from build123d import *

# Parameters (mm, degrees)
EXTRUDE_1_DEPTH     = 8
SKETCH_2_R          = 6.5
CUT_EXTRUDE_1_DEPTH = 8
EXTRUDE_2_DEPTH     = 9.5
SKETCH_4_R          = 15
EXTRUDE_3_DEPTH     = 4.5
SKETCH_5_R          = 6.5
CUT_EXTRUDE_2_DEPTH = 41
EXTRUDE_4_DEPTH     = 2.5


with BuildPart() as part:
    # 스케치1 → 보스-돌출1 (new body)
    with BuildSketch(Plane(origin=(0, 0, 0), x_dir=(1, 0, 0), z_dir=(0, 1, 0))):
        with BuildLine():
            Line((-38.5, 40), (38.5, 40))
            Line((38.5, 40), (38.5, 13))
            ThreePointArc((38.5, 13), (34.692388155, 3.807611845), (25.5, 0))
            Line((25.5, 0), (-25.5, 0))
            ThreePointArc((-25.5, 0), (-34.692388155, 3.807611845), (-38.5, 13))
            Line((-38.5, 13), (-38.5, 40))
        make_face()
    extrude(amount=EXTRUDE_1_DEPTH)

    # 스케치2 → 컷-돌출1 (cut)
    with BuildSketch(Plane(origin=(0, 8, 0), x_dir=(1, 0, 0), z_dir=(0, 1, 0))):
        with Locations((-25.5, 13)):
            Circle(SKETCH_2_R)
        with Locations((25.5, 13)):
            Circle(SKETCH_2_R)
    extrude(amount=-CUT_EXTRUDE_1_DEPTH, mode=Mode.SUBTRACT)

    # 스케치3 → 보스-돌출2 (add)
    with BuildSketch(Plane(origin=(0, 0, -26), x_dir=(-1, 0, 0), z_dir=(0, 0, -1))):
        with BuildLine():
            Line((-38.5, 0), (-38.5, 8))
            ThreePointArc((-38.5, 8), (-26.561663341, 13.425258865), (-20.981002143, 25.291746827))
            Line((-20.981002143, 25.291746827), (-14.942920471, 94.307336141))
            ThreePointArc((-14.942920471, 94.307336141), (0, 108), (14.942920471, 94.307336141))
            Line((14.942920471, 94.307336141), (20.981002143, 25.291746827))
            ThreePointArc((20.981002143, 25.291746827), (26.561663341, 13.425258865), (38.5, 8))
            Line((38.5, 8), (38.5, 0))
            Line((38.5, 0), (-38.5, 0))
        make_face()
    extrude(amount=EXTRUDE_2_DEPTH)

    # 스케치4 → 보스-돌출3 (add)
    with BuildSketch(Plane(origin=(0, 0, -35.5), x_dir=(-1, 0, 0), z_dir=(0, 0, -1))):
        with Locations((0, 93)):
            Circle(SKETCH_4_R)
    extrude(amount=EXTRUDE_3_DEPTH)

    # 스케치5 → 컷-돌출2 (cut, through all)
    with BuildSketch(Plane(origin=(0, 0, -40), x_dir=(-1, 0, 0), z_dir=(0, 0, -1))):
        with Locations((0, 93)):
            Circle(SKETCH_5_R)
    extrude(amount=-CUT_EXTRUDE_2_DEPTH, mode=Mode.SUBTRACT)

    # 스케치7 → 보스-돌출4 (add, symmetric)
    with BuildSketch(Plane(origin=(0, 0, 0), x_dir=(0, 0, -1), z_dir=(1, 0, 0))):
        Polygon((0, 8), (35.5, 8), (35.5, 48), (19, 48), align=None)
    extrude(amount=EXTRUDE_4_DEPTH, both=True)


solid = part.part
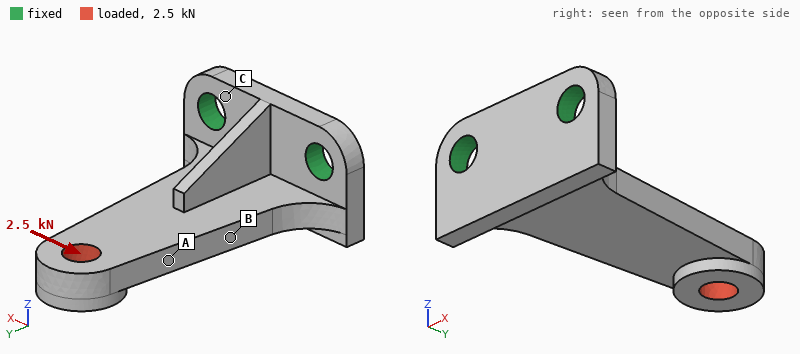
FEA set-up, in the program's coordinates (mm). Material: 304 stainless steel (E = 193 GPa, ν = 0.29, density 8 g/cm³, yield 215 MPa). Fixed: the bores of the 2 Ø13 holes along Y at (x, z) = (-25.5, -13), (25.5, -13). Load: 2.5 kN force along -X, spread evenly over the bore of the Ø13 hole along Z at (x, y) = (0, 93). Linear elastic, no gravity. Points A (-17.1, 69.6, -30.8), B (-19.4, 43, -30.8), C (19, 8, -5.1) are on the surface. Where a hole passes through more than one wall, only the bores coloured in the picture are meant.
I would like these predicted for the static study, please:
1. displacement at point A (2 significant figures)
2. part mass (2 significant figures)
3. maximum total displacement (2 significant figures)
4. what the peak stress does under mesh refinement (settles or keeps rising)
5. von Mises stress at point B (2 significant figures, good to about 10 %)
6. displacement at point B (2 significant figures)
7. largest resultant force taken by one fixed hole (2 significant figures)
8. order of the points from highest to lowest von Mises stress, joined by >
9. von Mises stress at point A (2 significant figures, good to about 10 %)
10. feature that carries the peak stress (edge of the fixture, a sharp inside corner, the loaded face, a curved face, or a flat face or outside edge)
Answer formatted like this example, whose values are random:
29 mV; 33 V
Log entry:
0.064 mm; 490 g; 0.12 mm; keeps rising; 54 MPa; 0.034 mm; 4.7 kN; B > A > C; 33 MPa; edge of the fixture
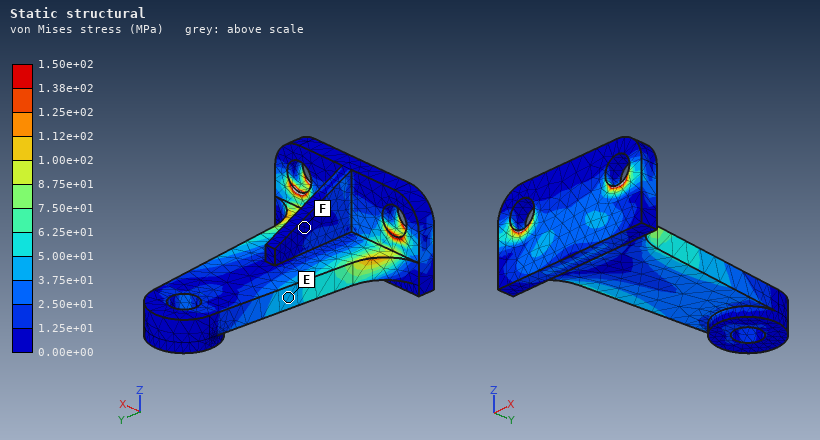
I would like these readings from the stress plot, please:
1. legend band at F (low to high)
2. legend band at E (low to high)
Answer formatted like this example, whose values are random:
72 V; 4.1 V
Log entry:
0.00e+00 to 1.25e+01 MPa; 3.75e+01 to 5.00e+01 MPa
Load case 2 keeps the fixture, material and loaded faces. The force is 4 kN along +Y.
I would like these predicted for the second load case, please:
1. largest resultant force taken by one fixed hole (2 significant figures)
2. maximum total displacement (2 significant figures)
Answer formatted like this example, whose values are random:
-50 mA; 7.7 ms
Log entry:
2.0 kN; 0.11 mm
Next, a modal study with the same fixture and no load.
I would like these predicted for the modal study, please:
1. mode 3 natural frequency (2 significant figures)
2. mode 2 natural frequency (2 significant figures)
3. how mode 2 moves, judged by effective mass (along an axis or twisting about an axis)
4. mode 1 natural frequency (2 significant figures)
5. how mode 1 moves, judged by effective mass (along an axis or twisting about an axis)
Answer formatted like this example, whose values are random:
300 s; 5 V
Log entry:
4000 Hz; 2500 Hz; along X; 1000 Hz; along Z
